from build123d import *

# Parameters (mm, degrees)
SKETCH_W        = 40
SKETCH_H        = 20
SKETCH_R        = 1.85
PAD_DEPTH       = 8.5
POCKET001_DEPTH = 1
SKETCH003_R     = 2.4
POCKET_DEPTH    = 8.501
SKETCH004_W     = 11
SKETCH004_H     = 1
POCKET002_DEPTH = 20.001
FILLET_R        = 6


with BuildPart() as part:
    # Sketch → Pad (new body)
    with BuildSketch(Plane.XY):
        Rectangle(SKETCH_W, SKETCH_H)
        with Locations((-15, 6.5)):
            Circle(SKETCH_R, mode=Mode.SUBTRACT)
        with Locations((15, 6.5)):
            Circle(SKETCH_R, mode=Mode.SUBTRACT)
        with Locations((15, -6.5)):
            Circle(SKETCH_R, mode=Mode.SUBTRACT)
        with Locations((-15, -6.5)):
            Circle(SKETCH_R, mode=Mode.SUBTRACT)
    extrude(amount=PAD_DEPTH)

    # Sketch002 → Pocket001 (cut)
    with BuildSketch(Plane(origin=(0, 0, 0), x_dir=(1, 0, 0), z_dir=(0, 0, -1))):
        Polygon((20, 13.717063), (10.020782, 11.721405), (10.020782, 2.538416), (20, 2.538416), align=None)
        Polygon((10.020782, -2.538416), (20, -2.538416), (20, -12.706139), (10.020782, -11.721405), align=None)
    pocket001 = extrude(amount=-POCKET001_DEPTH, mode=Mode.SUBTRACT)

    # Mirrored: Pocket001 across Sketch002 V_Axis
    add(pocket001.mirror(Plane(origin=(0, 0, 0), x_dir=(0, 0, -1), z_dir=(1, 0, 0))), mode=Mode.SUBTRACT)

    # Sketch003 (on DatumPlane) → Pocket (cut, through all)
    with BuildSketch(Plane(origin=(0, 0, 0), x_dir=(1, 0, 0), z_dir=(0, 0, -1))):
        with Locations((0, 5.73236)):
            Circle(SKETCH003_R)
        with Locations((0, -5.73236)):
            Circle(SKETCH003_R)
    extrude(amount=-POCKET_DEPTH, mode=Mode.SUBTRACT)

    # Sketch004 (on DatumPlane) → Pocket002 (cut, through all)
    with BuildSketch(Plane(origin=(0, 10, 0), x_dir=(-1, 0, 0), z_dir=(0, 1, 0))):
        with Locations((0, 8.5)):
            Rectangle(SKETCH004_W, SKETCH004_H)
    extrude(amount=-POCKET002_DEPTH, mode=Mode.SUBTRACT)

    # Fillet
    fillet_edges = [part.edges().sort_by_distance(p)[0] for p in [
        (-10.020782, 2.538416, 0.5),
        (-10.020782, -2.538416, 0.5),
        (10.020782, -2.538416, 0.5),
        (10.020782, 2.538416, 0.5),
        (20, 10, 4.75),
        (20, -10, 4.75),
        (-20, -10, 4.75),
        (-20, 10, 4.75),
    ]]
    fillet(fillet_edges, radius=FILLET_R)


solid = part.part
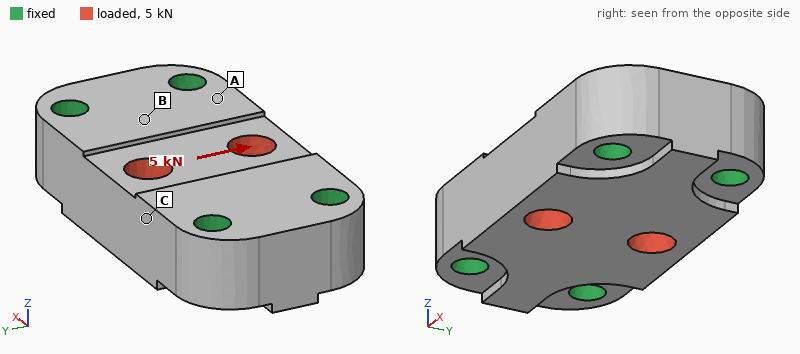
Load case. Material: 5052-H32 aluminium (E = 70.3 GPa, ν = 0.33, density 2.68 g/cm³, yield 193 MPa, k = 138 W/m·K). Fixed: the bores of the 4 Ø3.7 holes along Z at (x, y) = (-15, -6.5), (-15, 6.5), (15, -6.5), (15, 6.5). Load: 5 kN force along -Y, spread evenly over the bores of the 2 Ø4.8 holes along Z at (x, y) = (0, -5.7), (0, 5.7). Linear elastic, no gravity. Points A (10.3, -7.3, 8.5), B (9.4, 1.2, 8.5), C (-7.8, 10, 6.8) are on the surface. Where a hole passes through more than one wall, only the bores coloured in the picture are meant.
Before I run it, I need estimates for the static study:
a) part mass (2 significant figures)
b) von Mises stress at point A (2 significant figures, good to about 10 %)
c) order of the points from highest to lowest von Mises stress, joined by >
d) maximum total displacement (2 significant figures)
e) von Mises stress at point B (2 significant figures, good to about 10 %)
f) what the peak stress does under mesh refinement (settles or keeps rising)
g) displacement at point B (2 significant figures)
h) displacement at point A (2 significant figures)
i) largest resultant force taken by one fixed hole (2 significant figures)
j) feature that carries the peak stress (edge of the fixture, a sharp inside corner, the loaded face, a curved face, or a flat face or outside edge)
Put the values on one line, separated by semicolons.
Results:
15 g; 20 MPa; B > A > C; 13 µm; 36 MPa; keeps rising; 3.5 µm; 2.9 µm; 1.7 kN; edge of the fixture
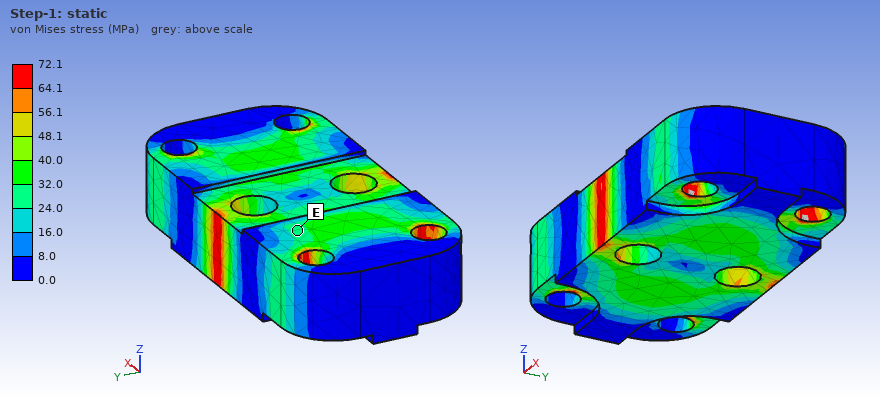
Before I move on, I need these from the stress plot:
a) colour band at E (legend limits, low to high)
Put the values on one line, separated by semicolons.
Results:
24.0 to 32.0 MPa
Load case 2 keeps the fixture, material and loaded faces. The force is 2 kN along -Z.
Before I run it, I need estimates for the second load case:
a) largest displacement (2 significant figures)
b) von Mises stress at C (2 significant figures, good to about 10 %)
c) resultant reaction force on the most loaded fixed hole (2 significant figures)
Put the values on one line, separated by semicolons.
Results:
10 µm; 15 MPa; 520 N
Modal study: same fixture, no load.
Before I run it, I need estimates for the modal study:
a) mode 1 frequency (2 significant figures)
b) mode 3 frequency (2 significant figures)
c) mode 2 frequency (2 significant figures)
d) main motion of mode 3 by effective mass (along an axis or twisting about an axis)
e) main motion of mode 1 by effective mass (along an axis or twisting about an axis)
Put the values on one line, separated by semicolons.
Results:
35 kHz; 50 kHz; 47 kHz; along Y; along Z
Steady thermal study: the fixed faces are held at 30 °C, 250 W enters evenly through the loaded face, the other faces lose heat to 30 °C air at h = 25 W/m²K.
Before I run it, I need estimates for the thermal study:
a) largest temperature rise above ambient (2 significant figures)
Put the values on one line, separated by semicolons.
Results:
83 K
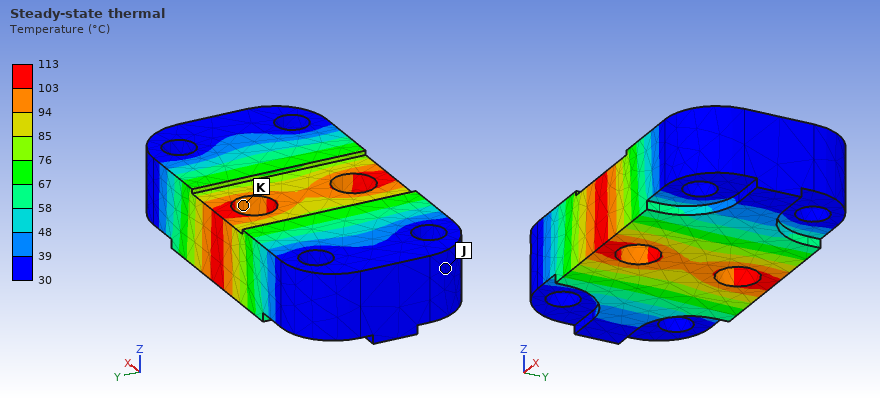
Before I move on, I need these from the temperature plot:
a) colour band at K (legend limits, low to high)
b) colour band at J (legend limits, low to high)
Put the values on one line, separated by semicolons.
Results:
94 to 103 °C; 30 to 39 °C
